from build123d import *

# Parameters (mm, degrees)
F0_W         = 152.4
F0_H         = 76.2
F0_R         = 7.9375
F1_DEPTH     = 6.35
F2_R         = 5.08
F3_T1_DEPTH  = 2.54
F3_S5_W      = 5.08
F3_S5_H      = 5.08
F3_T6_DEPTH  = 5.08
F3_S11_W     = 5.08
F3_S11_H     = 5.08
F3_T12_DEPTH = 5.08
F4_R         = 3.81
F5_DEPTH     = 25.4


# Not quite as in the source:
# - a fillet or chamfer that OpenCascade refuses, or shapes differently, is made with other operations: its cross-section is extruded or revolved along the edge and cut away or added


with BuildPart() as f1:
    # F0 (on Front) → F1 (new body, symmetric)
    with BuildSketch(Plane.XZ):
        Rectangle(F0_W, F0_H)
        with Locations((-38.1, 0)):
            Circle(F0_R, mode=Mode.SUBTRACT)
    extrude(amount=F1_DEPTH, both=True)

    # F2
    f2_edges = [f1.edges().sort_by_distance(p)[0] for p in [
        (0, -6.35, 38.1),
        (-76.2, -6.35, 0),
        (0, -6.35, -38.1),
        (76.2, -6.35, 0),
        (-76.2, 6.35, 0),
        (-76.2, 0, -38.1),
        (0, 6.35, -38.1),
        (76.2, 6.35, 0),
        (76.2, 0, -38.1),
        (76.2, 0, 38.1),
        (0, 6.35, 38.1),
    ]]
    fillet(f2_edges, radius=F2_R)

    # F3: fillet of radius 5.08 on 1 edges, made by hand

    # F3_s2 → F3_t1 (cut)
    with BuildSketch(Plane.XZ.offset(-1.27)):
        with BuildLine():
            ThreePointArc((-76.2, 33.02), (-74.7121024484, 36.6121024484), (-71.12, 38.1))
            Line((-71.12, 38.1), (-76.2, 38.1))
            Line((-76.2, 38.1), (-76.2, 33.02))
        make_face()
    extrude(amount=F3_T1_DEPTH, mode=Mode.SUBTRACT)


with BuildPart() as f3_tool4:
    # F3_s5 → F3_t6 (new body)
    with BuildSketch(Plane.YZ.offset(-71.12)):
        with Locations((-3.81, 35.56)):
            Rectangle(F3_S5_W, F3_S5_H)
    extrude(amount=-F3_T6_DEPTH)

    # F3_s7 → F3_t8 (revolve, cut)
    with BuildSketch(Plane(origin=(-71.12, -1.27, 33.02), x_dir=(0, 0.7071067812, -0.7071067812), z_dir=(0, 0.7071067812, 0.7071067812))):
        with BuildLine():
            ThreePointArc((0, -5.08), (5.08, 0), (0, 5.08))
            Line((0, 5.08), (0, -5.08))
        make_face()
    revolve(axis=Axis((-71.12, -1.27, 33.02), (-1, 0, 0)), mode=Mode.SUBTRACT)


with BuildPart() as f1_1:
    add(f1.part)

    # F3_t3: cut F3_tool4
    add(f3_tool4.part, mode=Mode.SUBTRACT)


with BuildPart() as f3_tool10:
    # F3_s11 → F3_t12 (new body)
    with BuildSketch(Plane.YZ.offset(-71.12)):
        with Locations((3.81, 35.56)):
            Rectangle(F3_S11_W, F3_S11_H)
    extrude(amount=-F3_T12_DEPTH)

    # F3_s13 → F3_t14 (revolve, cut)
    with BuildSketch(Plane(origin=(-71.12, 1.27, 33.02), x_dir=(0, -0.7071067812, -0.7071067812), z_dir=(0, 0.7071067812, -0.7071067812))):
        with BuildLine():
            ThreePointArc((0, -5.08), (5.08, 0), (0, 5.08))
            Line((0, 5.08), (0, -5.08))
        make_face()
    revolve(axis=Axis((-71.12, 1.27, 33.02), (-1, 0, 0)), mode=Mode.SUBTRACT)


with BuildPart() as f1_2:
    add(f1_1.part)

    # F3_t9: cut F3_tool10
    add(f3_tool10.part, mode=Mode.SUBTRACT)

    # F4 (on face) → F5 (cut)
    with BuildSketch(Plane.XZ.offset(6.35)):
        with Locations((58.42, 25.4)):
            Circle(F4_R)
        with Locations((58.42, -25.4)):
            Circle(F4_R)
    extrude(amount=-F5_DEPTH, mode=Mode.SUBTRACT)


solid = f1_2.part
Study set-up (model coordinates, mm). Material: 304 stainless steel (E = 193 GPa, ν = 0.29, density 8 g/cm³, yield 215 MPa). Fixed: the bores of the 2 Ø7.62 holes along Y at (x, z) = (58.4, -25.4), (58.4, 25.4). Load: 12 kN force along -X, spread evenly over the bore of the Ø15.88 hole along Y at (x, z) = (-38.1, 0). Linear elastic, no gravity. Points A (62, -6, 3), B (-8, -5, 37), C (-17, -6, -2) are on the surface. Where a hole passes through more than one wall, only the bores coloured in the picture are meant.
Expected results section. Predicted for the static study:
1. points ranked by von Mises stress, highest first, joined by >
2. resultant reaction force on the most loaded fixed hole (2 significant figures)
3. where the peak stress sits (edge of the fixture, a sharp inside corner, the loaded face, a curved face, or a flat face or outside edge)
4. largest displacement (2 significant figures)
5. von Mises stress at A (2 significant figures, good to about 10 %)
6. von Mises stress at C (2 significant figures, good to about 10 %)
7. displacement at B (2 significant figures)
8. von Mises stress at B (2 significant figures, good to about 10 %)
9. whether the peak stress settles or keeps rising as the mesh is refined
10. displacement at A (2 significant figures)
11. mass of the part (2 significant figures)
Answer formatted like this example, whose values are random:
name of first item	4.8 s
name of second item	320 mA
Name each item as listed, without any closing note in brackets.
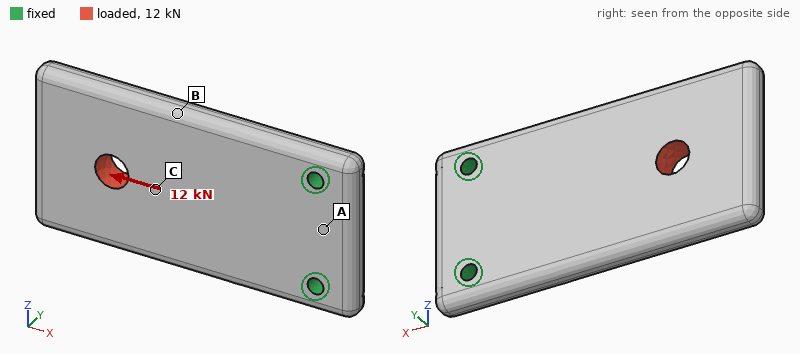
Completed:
points ranked by von Mises stress, highest first, joined by >	C > B > A
resultant reaction force on the most loaded fixed hole	6.0 kN
where the peak stress sits	edge of the fixture
largest displacement	9.2 µm
von Mises stress at A	3.0 MPa
von Mises stress at C	18 MPa
displacement at B	4.9 µm
von Mises stress at B	10 MPa
whether the peak stress settles or keeps rising as the mesh is refined	keeps rising
displacement at A	1.5 µm
mass of the part	1.1 kg
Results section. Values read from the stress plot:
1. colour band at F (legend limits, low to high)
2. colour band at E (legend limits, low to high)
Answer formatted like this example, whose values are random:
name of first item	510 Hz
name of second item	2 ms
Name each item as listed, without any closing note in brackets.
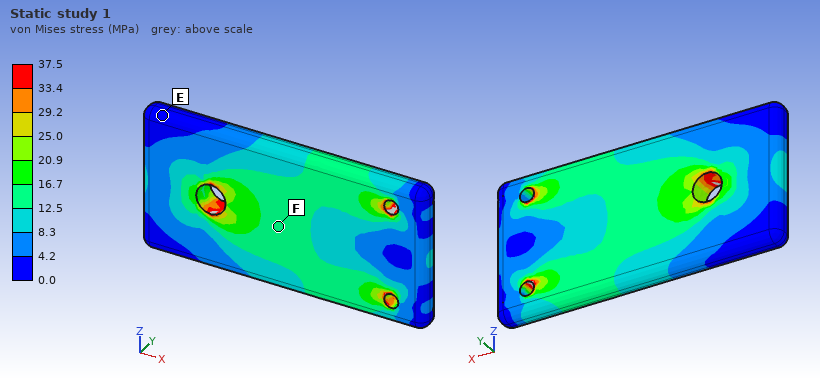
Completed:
colour band at F	12.5 to 16.7 MPa
colour band at E	0.0 to 4.2 MPa
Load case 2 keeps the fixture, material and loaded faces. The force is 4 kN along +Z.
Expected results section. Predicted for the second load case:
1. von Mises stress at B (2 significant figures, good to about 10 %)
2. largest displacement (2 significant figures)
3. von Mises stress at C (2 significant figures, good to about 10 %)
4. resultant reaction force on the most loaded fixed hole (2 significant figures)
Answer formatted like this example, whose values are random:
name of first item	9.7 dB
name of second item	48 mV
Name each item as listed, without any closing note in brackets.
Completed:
von Mises stress at B	10 MPa
largest displacement	32 µm
von Mises stress at C	12 MPa
resultant reaction force on the most loaded fixed hole	7.4 kN
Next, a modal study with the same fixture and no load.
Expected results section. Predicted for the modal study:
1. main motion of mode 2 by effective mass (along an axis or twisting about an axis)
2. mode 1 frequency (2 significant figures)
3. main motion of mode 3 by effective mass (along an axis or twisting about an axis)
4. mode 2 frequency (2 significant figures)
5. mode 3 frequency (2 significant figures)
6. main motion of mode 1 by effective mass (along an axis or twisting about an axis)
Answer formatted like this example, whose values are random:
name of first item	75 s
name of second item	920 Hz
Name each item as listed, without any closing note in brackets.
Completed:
main motion of mode 2 by effective mass	twisting about X
mode 1 frequency	550 Hz
main motion of mode 3 by effective mass	along Z
mode 2 frequency	2100 Hz
mode 3 frequency	2700 Hz
main motion of mode 1 by effective mass	along Y
